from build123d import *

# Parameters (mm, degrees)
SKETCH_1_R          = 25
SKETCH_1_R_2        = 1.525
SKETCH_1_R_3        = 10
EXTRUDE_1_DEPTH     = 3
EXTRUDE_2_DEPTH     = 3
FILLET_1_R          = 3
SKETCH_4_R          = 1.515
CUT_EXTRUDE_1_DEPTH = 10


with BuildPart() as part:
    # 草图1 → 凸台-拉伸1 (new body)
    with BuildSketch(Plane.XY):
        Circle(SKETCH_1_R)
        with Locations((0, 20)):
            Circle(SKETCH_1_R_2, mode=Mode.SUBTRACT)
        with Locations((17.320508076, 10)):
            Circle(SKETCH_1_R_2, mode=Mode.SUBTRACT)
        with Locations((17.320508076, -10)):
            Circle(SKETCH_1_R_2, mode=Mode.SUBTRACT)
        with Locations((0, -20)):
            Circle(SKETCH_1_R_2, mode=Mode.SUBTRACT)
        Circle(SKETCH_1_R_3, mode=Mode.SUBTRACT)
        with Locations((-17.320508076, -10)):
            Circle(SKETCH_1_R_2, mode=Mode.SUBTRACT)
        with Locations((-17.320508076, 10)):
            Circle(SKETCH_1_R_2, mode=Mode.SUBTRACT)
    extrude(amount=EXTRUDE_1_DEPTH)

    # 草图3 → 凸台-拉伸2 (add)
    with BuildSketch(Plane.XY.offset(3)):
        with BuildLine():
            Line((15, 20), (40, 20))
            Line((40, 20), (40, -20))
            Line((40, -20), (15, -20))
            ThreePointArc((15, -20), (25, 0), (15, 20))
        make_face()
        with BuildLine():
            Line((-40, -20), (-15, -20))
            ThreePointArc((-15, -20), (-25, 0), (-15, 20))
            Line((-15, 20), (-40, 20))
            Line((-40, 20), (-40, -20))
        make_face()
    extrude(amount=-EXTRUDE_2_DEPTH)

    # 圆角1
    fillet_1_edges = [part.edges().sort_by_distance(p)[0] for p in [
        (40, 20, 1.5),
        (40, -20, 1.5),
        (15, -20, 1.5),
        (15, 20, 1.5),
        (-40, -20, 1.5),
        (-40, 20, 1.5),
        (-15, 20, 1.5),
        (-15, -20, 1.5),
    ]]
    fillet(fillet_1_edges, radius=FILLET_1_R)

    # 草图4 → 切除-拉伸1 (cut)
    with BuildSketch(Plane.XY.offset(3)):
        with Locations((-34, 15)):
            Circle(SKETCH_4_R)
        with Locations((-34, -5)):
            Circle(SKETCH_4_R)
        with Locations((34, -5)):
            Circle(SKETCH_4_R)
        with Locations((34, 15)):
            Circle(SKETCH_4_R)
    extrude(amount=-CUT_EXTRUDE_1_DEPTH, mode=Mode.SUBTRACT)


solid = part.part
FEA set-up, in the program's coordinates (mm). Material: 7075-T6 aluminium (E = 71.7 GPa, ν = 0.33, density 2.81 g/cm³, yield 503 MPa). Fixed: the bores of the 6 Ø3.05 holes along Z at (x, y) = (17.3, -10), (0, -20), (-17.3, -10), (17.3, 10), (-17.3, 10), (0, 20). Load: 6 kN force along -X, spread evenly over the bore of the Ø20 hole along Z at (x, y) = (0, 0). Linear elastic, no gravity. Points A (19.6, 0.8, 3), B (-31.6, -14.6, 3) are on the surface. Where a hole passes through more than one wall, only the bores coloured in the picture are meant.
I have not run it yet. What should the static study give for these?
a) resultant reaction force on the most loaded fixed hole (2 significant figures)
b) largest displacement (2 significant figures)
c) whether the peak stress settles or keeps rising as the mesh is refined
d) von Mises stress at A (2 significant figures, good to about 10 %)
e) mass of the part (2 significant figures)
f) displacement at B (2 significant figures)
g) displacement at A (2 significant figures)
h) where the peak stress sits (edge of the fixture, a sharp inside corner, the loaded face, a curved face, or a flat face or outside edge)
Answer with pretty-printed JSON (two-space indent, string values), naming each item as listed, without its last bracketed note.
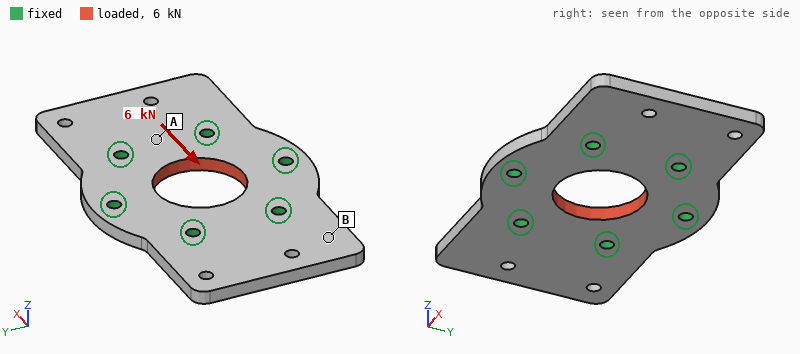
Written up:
{
  "resultant reaction force on the most loaded fixed hole": "1.3 kN",
  "largest displacement": "7.0 µm",
  "whether the peak stress settles or keeps rising as the mesh is refined": "keeps rising",
  "von Mises stress at A": "15 MPa",
  "mass of the part": "25 g",
  "displacement at B": "1.4 µm",
  "displacement at A": "3.3 µm",
  "where the peak stress sits": "edge of the fixture"
}
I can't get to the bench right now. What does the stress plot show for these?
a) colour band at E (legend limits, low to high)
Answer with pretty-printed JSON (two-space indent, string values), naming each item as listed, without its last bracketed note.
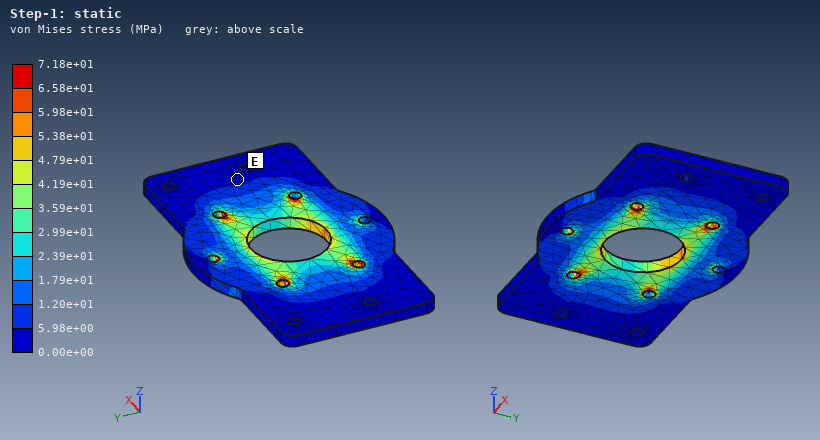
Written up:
{
  "colour band at E": "0.00e+00 to 5.98e+00 MPa"
}
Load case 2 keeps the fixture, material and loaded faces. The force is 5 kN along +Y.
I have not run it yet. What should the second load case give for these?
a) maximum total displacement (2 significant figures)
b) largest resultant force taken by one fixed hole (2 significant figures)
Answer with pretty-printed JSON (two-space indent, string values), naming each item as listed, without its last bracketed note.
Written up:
{
  "maximum total displacement": "5.8 µm",
  "largest resultant force taken by one fixed hole": "1.1 kN"
}
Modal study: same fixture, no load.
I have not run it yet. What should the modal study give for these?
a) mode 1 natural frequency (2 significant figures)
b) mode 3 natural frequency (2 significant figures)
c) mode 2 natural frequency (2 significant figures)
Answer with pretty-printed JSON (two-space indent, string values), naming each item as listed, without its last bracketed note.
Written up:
{
  "mode 1 natural frequency": "4700 Hz",
  "mode 3 natural frequency": "7300 Hz",
  "mode 2 natural frequency": "4700 Hz"
}
